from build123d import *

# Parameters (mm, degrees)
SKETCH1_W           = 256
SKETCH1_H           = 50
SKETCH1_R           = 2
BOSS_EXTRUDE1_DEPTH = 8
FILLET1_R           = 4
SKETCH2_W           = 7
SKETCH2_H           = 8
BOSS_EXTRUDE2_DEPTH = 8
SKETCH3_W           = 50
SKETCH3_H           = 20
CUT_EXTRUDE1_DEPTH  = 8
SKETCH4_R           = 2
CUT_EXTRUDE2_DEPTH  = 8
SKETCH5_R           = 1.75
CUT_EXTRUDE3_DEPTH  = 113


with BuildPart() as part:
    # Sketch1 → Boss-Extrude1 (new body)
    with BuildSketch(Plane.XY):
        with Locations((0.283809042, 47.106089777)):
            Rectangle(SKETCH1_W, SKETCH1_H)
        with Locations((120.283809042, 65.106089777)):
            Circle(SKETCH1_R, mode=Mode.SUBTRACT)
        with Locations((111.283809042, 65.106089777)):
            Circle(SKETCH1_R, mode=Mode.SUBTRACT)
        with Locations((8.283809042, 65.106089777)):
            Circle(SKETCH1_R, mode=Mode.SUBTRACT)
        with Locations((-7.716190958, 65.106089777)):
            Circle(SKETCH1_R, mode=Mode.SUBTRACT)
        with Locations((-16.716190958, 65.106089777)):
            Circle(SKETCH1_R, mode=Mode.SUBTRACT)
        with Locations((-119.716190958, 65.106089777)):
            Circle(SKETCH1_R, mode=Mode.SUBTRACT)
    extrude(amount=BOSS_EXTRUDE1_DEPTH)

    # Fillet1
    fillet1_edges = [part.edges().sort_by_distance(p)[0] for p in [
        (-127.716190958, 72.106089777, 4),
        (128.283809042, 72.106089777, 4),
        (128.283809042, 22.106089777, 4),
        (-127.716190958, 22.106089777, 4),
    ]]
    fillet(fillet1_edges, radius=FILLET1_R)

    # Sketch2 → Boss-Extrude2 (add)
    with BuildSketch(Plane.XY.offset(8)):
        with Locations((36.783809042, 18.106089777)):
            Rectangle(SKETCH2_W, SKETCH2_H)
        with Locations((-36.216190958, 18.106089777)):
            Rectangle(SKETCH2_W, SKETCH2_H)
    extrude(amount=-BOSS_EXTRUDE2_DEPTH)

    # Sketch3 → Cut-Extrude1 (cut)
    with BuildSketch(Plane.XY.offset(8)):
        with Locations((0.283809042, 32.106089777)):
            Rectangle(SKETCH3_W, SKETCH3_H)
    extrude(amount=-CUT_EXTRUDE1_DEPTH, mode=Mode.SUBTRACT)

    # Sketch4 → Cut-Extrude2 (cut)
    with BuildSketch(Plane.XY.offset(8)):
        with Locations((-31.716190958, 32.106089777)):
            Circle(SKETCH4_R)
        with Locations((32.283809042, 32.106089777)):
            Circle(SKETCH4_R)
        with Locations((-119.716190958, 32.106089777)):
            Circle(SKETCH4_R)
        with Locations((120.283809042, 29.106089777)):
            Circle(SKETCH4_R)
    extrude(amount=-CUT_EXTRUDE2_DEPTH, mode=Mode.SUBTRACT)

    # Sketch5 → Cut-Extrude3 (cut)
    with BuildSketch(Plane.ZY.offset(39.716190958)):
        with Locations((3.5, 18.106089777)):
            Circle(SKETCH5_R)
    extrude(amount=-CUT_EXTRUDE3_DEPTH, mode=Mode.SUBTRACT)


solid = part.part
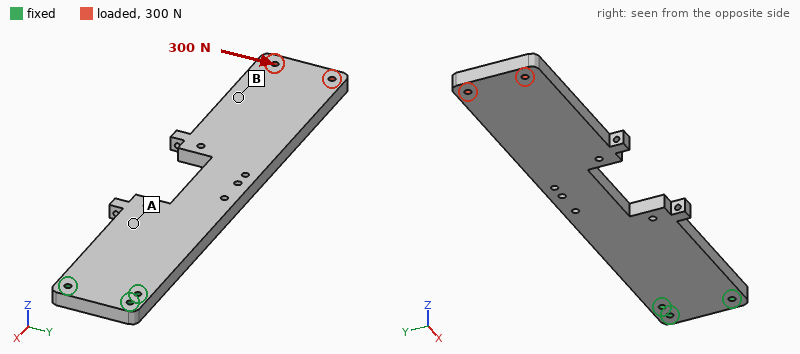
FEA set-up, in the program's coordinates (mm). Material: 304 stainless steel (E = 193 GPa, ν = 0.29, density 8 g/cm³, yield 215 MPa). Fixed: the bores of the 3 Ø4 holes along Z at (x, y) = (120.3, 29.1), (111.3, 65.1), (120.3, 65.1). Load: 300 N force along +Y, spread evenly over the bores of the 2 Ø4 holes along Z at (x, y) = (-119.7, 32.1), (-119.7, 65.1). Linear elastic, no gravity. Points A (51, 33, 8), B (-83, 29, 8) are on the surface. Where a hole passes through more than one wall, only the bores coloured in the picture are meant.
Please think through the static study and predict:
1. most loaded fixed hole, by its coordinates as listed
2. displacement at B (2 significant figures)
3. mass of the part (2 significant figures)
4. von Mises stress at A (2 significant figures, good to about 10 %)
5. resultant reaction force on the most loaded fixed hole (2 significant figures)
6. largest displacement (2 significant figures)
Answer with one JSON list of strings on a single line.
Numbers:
["(120.3, 29.1)", "0.12 mm", "750 g", "11 MPa", "1.8 kN", "0.18 mm"]
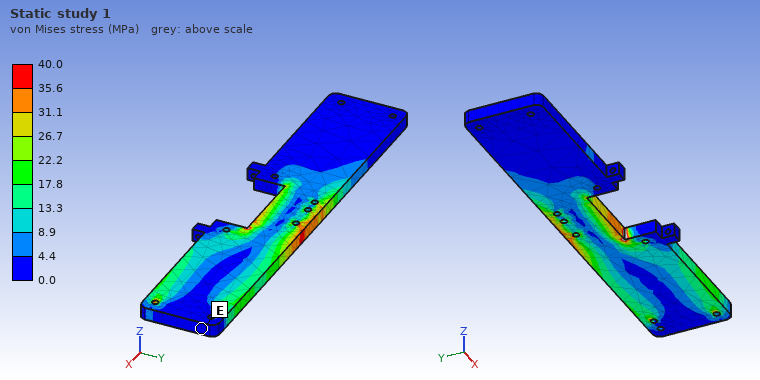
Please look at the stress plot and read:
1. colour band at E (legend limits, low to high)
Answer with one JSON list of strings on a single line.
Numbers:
["0.0 to 4.4 MPa"]
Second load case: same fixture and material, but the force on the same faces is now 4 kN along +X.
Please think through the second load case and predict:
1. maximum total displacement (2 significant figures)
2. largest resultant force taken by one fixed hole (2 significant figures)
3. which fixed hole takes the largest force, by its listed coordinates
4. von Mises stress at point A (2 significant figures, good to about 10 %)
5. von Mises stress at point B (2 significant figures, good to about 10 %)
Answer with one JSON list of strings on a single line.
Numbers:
["95 µm", "1.8 kN", "(120.3, 29.1)", "10.0 MPa", "8.8 MPa"]
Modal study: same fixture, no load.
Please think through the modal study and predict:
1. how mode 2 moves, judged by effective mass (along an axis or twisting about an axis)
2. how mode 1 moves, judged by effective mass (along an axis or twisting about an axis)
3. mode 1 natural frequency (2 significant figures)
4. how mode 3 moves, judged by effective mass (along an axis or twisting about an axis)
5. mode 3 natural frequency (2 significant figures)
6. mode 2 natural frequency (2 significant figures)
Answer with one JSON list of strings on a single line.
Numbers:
["along Y", "along Z", "100 Hz", "along Z", "640 Hz", "500 Hz"]
